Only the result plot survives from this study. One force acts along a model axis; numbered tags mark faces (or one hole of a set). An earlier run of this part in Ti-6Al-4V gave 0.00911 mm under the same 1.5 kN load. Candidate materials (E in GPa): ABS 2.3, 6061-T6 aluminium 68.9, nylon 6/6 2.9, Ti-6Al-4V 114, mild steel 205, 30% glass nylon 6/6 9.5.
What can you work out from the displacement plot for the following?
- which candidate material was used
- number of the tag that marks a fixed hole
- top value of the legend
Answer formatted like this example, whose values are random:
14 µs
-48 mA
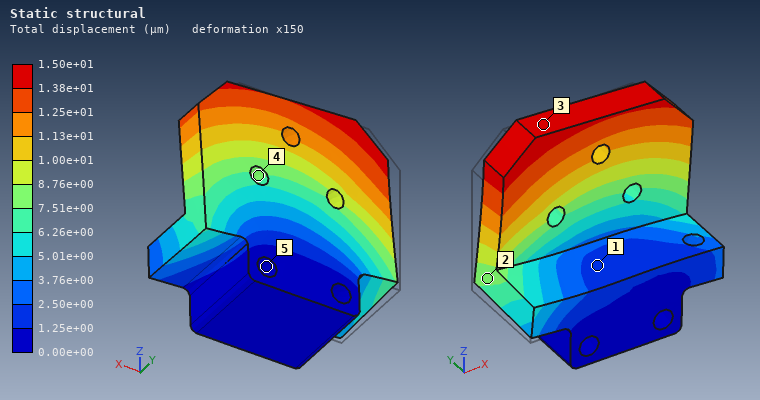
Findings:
6061-T6 aluminium
5
1.50e+01 µm
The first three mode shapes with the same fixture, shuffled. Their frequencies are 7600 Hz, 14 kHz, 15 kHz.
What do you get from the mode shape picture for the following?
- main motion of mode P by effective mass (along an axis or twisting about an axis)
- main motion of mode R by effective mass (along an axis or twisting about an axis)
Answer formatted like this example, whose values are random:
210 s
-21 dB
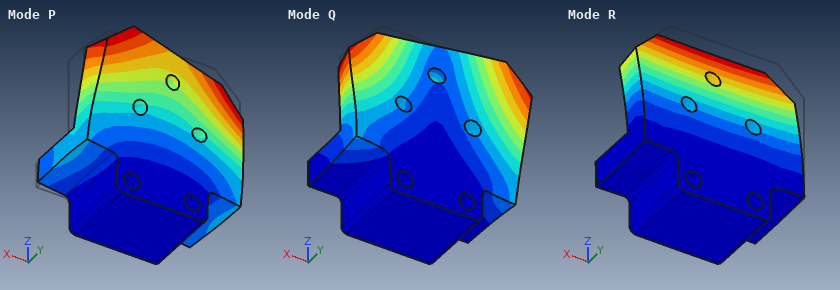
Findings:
along X
along Y
